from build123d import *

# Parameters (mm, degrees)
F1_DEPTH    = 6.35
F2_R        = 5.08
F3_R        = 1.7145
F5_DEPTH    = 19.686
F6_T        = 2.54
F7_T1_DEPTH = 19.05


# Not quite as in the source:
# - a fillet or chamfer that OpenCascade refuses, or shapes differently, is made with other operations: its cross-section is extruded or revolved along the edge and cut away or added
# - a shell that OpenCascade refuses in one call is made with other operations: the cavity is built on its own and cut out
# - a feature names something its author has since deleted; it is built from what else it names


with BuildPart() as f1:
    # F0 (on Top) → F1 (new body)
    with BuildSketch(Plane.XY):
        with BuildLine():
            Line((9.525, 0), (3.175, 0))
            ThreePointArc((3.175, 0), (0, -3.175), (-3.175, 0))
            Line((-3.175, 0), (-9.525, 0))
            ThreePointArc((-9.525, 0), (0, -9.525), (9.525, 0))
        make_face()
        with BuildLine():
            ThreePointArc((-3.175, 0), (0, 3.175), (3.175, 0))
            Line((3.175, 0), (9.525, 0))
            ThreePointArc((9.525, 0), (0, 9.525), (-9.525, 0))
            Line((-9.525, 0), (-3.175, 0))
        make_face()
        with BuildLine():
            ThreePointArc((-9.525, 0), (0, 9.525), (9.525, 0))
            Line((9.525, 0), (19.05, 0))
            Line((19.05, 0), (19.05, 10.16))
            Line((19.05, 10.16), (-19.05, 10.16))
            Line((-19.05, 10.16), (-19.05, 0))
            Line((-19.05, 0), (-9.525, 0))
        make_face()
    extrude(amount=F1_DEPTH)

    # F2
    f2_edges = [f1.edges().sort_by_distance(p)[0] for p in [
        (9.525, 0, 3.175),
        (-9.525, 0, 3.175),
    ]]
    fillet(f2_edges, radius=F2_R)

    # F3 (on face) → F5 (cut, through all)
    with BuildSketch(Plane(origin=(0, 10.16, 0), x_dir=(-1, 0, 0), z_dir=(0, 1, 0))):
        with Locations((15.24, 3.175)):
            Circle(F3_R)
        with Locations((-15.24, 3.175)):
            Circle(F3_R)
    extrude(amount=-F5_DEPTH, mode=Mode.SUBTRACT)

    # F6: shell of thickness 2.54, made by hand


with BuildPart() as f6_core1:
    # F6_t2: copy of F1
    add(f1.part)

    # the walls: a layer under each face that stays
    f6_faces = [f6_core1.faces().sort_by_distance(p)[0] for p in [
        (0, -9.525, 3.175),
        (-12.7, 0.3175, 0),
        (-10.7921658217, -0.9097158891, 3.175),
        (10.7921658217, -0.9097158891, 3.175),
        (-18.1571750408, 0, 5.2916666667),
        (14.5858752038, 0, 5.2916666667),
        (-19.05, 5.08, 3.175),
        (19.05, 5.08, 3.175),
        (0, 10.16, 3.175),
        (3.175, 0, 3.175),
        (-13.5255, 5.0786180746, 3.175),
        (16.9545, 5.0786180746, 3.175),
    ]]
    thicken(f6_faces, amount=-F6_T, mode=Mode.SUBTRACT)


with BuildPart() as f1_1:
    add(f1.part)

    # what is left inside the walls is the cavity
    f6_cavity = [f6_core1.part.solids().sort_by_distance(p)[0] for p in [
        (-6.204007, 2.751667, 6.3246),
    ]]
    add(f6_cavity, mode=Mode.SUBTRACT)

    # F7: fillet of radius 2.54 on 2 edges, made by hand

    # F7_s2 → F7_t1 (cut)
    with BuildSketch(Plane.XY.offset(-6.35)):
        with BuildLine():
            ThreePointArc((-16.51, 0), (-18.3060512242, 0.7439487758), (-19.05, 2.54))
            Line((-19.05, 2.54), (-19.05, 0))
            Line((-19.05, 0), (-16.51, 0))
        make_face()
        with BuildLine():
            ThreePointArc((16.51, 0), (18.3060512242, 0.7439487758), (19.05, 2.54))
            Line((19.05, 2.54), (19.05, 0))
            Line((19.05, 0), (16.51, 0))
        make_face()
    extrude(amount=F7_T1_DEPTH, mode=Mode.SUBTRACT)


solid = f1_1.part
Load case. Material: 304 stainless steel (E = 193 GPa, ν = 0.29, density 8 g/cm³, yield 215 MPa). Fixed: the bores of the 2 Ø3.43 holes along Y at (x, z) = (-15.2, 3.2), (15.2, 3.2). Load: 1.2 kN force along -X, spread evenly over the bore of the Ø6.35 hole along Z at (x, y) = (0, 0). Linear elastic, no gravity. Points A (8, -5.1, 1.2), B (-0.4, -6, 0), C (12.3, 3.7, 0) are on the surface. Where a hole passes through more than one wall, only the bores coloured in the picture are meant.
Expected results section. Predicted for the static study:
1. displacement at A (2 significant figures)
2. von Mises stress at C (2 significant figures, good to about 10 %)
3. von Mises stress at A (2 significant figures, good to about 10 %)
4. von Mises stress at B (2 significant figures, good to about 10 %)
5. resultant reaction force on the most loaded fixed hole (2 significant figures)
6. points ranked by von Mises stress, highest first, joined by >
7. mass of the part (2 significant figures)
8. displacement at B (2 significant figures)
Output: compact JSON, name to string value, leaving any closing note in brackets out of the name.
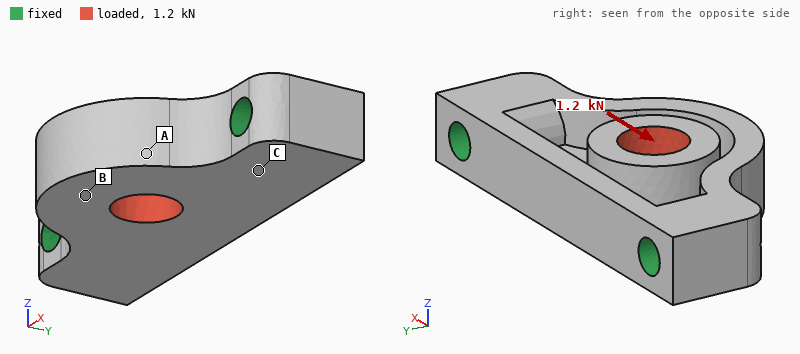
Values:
{"displacement at A": "1.8 µm", "von Mises stress at C": "21 MPa", "von Mises stress at A": "13 MPa", "von Mises stress at B": "4.8 MPa", "resultant reaction force on the most loaded fixed hole": "630 N", "points ranked by von Mises stress, highest first, joined by >": "C > A > B", "mass of the part": "20 g", "displacement at B": "1.2 µm"}
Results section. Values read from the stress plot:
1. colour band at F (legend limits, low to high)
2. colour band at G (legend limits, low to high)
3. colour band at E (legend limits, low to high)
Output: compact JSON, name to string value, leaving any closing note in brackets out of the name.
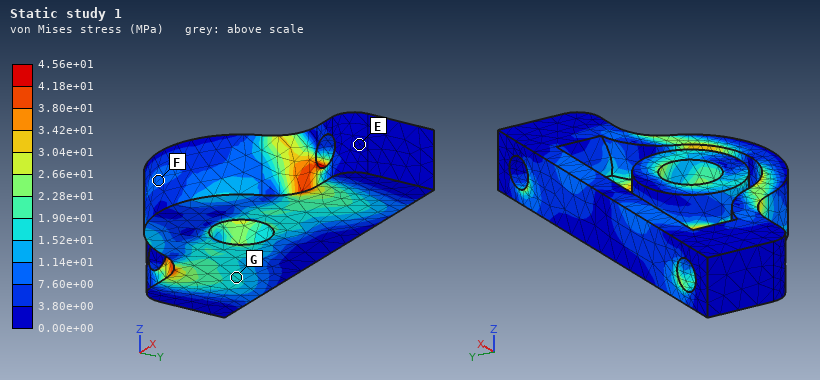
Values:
{"colour band at F": "7.60e+00 to 1.14e+01 MPa", "colour band at G": "1.52e+01 to 1.90e+01 MPa", "colour band at E": "0.00e+00 to 3.80e+00 MPa"}
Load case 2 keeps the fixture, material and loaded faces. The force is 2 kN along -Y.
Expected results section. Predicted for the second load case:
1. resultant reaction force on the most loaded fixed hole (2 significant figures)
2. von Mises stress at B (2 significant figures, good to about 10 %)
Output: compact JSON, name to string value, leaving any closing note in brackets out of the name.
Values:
{"resultant reaction force on the most loaded fixed hole": "1.1 kN", "von Mises stress at B": "48 MPa"}
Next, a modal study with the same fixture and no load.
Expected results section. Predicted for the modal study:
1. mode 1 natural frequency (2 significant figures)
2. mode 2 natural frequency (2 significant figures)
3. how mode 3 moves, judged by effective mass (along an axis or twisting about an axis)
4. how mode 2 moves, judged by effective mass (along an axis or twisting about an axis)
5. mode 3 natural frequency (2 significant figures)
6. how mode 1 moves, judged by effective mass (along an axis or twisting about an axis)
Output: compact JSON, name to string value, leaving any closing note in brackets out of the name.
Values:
{"mode 1 natural frequency": "15 kHz", "mode 2 natural frequency": "27 kHz", "how mode 3 moves, judged by effective mass": "along Y", "how mode 2 moves, judged by effective mass": "along Z", "mode 3 natural frequency": "34 kHz", "how mode 1 moves, judged by effective mass": "along Z"}
